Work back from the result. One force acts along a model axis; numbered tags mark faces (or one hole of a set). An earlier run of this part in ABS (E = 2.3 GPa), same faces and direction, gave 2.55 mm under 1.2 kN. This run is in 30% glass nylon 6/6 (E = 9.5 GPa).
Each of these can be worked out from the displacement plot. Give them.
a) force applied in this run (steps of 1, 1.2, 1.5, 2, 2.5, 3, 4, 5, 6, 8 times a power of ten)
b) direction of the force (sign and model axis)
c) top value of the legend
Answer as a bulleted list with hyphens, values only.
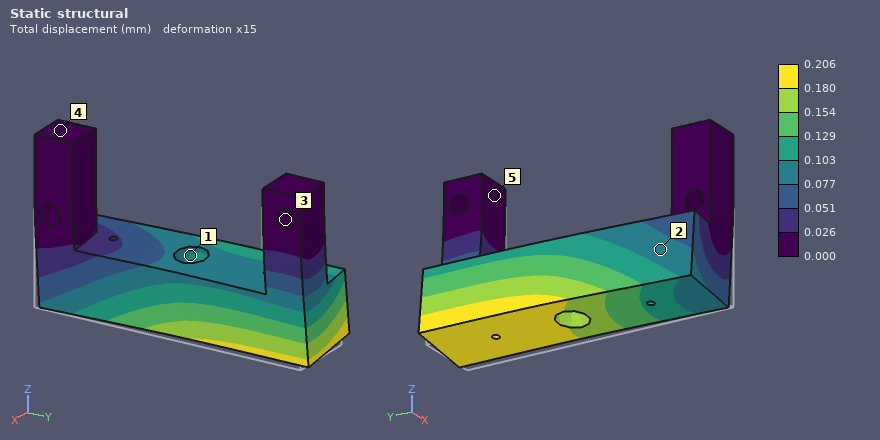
- 400 N
- -X
- 0.206 mm
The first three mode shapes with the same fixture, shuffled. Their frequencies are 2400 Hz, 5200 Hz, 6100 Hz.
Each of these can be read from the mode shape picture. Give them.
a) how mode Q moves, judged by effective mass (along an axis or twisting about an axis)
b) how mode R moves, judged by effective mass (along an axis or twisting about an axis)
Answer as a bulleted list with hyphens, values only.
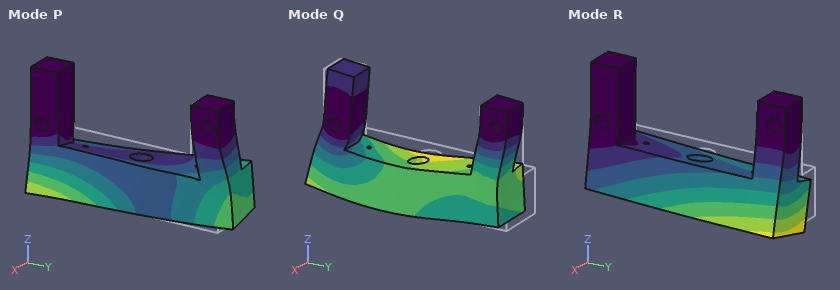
- along Y
- along X
